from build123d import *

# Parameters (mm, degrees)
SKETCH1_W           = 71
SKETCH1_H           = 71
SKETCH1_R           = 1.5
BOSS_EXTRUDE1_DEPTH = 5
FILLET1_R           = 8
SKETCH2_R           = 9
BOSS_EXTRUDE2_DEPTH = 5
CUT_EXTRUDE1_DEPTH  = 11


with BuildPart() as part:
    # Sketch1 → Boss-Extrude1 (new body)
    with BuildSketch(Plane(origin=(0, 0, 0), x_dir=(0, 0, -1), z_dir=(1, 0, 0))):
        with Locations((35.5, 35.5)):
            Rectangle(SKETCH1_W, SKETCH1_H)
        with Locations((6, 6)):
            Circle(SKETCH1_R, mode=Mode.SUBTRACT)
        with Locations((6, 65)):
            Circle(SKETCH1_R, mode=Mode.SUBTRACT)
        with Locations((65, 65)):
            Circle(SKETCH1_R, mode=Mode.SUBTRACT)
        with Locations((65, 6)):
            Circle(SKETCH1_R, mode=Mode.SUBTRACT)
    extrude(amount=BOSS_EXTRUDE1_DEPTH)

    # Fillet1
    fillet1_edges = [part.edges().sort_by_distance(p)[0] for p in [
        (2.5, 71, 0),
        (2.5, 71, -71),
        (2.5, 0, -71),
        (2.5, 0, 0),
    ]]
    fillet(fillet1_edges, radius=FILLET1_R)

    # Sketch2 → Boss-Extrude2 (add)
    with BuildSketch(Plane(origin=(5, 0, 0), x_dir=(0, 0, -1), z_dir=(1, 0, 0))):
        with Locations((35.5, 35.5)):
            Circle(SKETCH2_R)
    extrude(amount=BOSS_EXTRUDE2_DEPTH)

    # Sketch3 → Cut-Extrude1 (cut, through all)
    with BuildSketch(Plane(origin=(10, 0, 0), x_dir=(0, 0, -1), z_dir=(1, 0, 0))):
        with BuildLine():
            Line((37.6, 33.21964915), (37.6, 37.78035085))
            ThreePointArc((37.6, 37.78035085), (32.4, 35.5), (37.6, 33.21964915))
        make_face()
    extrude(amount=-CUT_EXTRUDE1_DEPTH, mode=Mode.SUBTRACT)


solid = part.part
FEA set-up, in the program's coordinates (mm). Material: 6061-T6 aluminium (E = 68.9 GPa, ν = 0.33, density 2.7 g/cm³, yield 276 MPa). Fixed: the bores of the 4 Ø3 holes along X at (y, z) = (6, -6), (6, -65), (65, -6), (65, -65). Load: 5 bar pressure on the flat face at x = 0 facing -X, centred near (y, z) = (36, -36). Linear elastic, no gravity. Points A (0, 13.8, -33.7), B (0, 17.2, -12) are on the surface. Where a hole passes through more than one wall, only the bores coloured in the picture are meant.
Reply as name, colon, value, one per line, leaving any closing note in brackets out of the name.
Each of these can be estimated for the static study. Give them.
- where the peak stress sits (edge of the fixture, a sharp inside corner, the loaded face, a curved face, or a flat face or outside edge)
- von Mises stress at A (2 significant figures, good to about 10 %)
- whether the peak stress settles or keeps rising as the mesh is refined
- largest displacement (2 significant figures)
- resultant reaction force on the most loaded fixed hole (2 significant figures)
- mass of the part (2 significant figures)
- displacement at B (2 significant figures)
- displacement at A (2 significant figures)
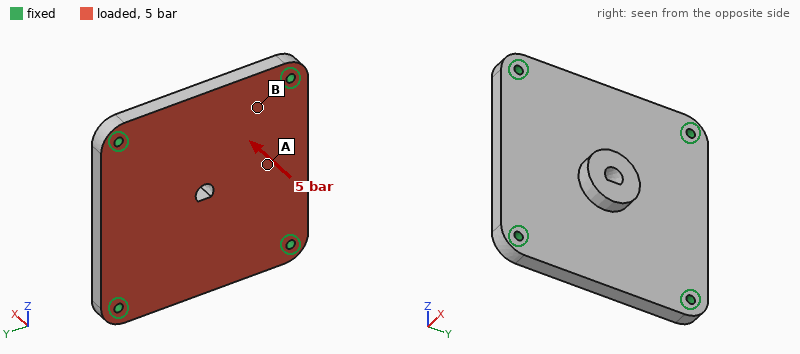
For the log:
where the peak stress sits: edge of the fixture
von Mises stress at A: 21 MPa
whether the peak stress settles or keeps rising as the mesh is refined: keeps rising
largest displacement: 60 µm
resultant reaction force on the most loaded fixed hole: 620 N
mass of the part: 70 g
displacement at B: 26 µm
displacement at A: 47 µm
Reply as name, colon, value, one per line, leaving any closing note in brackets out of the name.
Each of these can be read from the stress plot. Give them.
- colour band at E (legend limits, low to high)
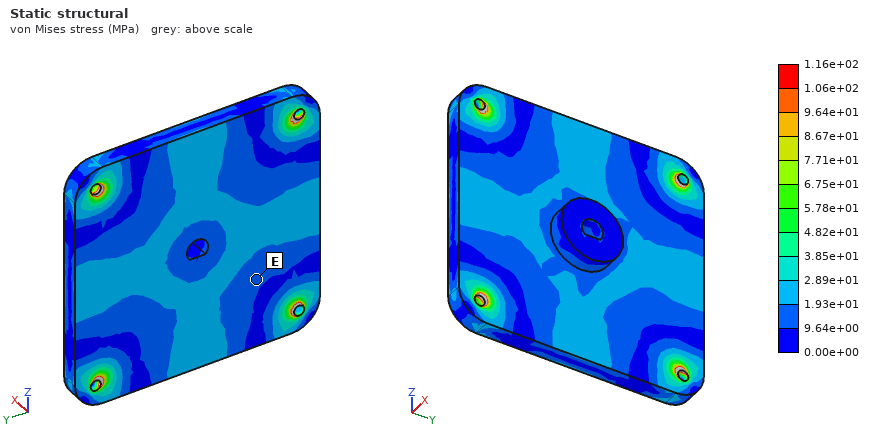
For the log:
colour band at E: 9.64e+00 to 1.93e+01 MPa
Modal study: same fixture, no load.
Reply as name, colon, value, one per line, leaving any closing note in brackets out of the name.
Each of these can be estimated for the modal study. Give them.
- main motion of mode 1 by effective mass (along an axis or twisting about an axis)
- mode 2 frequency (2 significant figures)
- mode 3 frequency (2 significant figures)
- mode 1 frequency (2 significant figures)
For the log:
main motion of mode 1 by effective mass: along X
mode 2 frequency: 7500 Hz
mode 3 frequency: 7500 Hz
mode 1 frequency: 4400 Hz
